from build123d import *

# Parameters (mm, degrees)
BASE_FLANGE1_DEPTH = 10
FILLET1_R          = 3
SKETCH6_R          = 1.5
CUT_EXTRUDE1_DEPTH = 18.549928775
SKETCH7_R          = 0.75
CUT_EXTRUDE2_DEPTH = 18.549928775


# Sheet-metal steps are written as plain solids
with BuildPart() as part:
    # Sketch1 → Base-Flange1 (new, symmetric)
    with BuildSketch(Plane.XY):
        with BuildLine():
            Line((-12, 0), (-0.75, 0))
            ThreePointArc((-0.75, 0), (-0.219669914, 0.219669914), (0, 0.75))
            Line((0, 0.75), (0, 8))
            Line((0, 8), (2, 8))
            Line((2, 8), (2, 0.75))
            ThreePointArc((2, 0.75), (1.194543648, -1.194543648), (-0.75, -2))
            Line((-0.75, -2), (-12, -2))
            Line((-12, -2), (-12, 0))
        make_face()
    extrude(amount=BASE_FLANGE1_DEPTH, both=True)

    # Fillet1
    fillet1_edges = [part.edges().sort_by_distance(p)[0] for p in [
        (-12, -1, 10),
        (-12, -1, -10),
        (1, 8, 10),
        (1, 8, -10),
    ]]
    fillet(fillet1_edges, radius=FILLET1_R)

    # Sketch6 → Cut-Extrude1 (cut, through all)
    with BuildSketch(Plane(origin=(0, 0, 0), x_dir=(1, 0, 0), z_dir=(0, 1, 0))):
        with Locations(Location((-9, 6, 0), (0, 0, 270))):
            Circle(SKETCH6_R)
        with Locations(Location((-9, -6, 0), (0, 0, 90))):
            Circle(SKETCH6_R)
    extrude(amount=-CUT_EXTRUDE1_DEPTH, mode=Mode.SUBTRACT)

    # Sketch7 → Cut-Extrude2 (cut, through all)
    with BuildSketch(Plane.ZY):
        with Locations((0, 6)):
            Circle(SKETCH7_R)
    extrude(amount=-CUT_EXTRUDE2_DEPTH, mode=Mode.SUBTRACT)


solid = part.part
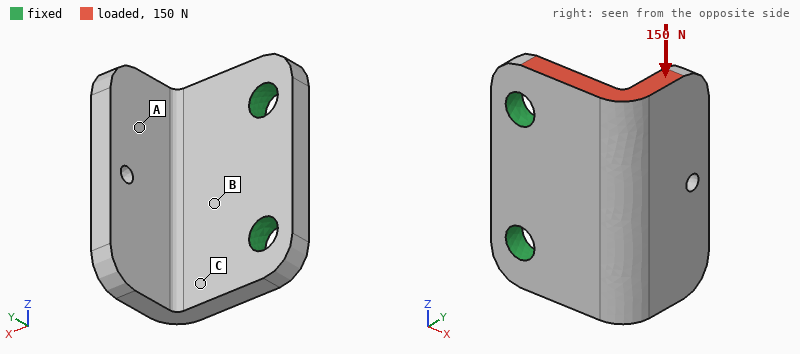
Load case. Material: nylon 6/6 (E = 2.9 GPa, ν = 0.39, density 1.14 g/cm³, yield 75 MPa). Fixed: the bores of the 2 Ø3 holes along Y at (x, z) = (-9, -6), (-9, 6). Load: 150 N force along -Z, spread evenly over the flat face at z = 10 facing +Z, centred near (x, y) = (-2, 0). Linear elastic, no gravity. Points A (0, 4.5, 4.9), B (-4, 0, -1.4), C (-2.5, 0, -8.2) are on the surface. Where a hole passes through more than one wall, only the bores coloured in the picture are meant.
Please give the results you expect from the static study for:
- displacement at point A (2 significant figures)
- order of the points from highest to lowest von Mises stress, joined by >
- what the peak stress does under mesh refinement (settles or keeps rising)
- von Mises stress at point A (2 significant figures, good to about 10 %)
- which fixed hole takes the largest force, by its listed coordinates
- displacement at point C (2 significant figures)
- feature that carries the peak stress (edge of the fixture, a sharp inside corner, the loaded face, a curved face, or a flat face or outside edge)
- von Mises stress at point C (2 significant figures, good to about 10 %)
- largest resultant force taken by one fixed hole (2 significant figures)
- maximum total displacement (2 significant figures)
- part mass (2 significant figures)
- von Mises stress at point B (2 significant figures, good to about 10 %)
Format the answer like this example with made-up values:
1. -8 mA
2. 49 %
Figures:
1. 0.12 mm
2. B > C > A
3. keeps rising
4. 2.9 MPa
5. (-9, 6)
6. 0.058 mm
7. edge of the fixture
8. 6.8 MPa
9. 110 N
10. 0.17 mm
11. 0.92 g
12. 11 MPa
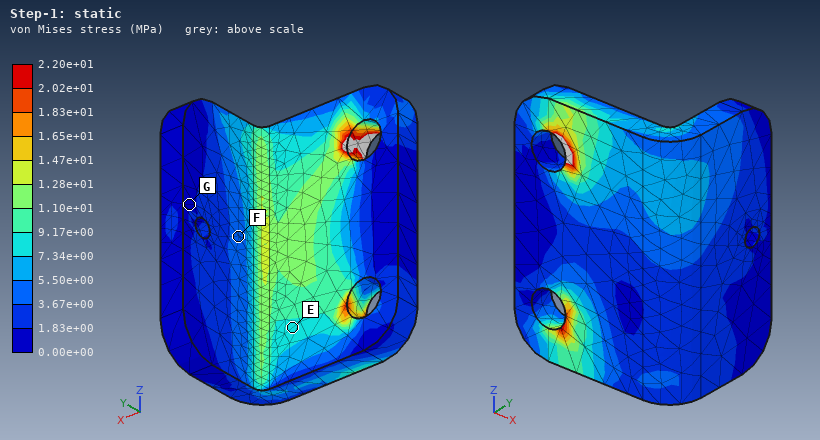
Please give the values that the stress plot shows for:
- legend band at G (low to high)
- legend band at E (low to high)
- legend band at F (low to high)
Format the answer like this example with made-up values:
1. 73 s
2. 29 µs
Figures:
1. 0.00e+00 to 1.83e+00 MPa
2. 7.34e+00 to 9.17e+00 MPa
3. 3.67e+00 to 5.50e+00 MPa
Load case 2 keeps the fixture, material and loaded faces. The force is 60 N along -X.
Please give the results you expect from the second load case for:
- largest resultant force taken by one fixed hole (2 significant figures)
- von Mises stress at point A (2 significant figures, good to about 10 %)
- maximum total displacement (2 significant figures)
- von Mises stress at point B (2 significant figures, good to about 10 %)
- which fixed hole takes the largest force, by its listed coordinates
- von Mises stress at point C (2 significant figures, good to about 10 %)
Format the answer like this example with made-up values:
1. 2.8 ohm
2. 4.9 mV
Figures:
1. 73 N
2. 5.1 MPa
3. 0.27 mm
4. 3.4 MPa
5. (-9, 6)
6. 2.2 MPa
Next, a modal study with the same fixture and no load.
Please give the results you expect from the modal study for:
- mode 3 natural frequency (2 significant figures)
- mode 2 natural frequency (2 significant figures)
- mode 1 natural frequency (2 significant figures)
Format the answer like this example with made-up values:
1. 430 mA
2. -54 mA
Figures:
1. 6300 Hz
2. 3700 Hz
3. 2200 Hz
